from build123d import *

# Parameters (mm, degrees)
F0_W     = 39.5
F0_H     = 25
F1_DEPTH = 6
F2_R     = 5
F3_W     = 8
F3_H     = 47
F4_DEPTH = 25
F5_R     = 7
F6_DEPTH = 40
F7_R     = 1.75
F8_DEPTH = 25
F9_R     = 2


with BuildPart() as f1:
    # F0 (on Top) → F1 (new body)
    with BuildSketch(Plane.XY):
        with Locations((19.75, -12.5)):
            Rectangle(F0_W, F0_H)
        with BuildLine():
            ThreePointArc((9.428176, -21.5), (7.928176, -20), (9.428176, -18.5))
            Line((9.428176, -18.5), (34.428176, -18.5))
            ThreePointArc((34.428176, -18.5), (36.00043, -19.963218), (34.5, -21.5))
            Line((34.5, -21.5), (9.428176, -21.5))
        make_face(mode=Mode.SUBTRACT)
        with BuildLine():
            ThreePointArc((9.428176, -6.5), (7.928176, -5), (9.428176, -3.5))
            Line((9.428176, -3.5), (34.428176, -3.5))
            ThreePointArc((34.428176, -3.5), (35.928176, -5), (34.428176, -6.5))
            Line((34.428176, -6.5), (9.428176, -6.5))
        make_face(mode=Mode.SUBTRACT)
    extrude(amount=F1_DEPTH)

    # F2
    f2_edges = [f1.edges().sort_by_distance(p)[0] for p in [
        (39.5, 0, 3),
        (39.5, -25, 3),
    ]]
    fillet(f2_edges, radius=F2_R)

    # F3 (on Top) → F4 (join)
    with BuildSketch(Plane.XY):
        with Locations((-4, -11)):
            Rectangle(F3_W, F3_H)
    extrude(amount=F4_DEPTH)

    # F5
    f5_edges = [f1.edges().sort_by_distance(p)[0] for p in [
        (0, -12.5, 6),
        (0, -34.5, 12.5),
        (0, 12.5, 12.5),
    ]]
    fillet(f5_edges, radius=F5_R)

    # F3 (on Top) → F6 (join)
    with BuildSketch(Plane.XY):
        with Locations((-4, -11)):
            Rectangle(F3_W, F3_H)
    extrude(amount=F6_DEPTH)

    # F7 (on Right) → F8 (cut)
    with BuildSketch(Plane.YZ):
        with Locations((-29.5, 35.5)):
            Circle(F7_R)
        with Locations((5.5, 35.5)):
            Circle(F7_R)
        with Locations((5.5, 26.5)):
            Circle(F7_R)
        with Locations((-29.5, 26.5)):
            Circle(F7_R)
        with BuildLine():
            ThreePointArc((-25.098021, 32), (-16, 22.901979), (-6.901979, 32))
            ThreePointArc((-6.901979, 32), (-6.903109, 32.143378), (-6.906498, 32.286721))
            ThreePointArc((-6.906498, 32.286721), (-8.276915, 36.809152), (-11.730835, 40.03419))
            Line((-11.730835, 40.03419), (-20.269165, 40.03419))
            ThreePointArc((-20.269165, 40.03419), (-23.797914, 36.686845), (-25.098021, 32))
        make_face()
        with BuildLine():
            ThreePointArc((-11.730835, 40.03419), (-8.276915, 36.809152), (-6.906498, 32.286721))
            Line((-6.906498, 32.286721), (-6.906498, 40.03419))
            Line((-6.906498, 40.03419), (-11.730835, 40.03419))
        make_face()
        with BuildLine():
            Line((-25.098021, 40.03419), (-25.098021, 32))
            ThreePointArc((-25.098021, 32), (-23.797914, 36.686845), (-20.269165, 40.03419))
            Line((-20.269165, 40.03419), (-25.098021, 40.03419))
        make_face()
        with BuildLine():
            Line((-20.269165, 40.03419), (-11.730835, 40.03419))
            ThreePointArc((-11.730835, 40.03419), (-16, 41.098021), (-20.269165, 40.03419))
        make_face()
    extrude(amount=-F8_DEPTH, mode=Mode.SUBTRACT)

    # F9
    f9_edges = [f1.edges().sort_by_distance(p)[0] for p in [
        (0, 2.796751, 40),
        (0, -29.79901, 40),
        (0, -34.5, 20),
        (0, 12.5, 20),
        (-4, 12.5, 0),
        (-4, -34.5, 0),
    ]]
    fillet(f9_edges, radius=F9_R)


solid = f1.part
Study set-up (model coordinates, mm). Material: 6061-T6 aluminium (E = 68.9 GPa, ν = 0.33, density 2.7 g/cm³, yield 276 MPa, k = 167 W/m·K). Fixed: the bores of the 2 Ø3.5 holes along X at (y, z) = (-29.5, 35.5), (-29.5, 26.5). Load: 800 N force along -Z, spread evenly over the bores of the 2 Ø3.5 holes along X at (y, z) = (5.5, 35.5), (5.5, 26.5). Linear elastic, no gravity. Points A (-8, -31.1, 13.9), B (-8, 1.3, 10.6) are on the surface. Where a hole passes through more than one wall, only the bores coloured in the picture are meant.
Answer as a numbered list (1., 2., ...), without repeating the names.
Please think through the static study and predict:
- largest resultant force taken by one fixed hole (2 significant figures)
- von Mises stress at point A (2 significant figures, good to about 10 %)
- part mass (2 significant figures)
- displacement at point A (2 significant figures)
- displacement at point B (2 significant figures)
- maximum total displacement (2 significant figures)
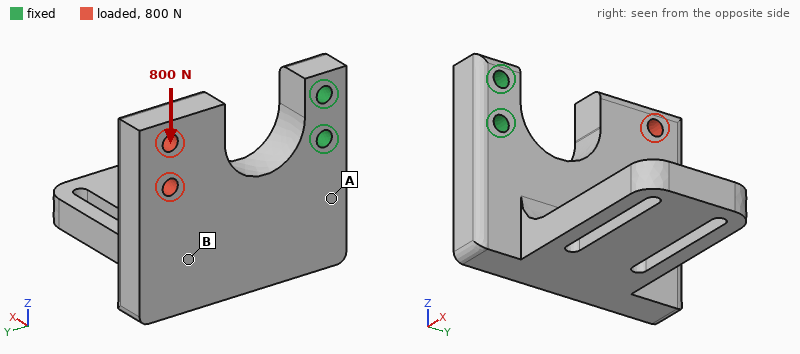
1. 1.5 kN
2. 32 MPa
3. 47 g
4. 0.048 mm
5. 0.16 mm
6. 0.23 mm
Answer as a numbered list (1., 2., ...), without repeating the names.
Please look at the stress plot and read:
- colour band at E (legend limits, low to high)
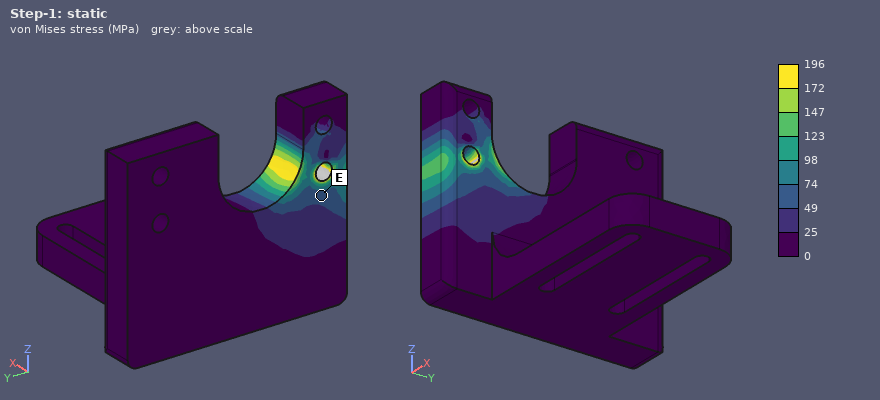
1. 49 to 74 MPa
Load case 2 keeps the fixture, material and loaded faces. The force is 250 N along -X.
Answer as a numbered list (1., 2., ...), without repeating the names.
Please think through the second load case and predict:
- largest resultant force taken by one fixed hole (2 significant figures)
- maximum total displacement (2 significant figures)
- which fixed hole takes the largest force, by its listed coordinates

1. 230 N
2. 0.16 mm
3. (-29.5, 26.5)
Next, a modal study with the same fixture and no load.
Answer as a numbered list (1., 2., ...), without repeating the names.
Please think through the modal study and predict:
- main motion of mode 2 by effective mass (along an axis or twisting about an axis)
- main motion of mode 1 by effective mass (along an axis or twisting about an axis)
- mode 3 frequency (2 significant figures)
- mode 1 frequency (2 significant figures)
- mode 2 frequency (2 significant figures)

1. along Z
2. along X
3. 2400 Hz
4. 1500 Hz
5. 1700 Hz
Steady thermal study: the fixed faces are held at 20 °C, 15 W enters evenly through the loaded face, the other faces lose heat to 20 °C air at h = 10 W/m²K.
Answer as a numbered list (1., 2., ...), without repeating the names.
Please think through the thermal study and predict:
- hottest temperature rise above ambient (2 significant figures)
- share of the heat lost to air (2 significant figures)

1. 27 K
2. 6.5 %
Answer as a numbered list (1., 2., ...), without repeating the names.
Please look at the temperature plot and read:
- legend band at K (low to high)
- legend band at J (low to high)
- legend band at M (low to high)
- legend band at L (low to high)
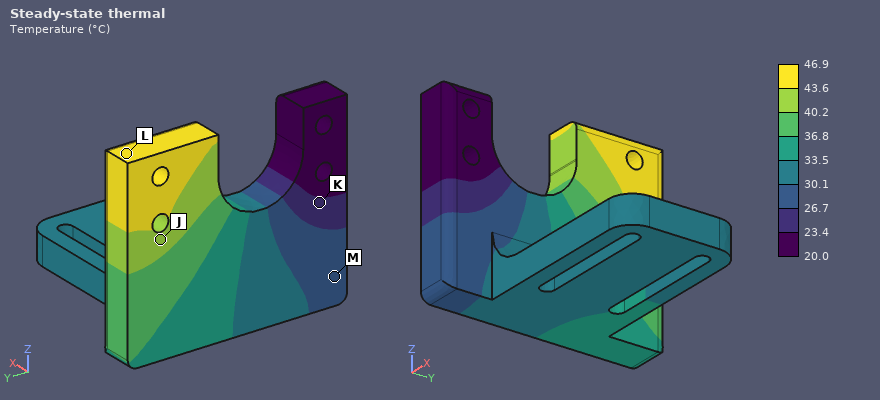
1. 23.4 to 26.7 °C
2. 40.2 to 43.6 °C
3. 26.7 to 30.1 °C
4. 43.6 to 46.9 °C
